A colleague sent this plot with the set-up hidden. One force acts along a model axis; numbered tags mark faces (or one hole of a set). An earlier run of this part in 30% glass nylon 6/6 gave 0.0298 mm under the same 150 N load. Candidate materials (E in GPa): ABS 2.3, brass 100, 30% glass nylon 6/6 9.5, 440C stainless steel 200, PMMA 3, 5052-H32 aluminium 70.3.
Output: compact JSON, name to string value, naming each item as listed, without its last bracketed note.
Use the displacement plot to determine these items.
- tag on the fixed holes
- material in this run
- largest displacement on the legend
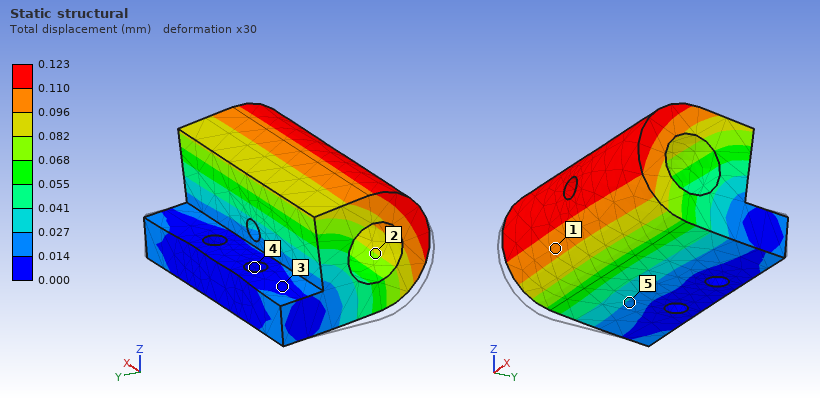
{"tag on the fixed holes": "4", "material in this run": "ABS", "largest displacement on the legend": "0.123 mm"}
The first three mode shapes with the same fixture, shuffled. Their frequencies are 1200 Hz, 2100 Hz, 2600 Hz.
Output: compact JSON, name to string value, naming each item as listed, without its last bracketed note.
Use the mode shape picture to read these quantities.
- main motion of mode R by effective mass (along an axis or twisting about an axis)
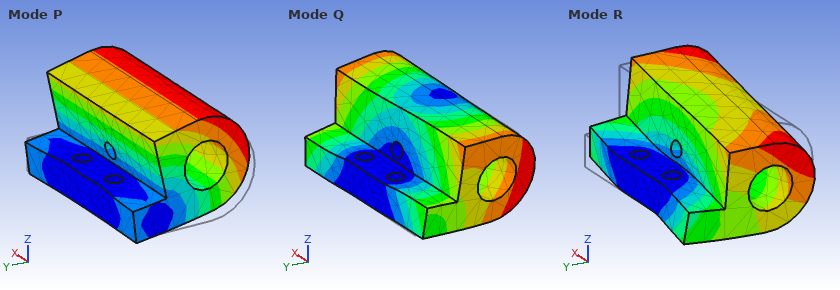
{"main motion of mode R by effective mass": "along X"}
